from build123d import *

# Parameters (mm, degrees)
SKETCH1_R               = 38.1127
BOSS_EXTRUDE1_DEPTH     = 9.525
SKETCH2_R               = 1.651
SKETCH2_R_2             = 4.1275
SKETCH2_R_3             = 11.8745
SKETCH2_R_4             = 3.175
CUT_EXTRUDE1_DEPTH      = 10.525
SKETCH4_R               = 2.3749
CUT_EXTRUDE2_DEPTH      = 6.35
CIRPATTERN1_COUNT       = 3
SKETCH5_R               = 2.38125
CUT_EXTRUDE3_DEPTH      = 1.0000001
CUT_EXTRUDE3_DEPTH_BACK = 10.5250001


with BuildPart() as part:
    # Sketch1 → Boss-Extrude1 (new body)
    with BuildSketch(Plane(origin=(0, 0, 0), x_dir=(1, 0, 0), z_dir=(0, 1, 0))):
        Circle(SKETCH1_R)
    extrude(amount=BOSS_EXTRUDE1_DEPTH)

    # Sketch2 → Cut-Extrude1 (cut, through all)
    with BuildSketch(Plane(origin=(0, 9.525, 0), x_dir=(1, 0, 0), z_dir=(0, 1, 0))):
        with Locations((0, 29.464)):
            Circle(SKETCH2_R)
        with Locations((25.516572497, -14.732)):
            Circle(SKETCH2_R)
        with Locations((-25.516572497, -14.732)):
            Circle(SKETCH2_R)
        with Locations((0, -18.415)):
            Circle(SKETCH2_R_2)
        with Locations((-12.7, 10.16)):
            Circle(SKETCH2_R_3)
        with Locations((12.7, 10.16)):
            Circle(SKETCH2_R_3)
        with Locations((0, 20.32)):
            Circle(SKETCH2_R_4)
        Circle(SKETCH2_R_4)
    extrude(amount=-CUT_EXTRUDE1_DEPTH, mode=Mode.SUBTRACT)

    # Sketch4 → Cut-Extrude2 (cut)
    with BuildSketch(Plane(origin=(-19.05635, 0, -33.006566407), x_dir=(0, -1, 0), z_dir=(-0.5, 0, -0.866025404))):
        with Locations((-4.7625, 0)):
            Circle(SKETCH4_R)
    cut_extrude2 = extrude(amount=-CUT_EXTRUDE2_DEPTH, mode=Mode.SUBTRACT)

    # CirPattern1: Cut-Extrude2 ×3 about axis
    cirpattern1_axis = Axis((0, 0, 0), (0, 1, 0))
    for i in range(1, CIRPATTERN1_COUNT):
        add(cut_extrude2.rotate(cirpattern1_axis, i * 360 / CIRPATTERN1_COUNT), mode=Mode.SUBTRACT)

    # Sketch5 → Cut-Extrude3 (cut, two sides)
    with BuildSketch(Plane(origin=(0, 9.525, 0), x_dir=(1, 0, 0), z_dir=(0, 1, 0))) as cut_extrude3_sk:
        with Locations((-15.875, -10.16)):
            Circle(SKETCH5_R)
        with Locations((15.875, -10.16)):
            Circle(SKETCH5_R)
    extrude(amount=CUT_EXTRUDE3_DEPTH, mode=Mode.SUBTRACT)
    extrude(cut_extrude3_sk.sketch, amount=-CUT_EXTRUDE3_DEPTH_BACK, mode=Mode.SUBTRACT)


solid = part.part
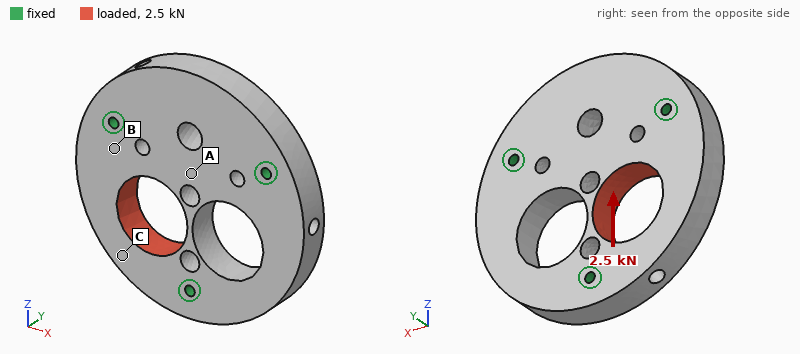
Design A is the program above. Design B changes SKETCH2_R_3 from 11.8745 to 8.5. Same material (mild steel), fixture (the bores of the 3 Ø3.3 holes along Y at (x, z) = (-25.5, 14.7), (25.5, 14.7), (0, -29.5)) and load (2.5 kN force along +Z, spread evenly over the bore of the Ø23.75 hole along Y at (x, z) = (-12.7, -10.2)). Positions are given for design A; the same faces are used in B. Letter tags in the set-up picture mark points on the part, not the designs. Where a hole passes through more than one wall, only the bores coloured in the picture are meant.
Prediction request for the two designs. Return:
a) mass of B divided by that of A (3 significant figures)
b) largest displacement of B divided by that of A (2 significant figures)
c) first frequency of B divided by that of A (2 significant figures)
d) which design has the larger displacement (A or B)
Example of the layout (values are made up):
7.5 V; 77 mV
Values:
1.12; 0.73; 1.0; A
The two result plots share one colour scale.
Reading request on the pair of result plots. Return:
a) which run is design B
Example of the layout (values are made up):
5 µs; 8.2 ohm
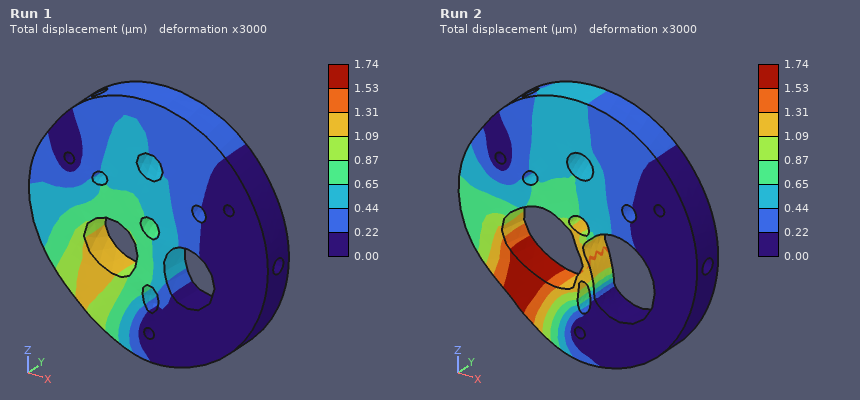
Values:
Run 1
